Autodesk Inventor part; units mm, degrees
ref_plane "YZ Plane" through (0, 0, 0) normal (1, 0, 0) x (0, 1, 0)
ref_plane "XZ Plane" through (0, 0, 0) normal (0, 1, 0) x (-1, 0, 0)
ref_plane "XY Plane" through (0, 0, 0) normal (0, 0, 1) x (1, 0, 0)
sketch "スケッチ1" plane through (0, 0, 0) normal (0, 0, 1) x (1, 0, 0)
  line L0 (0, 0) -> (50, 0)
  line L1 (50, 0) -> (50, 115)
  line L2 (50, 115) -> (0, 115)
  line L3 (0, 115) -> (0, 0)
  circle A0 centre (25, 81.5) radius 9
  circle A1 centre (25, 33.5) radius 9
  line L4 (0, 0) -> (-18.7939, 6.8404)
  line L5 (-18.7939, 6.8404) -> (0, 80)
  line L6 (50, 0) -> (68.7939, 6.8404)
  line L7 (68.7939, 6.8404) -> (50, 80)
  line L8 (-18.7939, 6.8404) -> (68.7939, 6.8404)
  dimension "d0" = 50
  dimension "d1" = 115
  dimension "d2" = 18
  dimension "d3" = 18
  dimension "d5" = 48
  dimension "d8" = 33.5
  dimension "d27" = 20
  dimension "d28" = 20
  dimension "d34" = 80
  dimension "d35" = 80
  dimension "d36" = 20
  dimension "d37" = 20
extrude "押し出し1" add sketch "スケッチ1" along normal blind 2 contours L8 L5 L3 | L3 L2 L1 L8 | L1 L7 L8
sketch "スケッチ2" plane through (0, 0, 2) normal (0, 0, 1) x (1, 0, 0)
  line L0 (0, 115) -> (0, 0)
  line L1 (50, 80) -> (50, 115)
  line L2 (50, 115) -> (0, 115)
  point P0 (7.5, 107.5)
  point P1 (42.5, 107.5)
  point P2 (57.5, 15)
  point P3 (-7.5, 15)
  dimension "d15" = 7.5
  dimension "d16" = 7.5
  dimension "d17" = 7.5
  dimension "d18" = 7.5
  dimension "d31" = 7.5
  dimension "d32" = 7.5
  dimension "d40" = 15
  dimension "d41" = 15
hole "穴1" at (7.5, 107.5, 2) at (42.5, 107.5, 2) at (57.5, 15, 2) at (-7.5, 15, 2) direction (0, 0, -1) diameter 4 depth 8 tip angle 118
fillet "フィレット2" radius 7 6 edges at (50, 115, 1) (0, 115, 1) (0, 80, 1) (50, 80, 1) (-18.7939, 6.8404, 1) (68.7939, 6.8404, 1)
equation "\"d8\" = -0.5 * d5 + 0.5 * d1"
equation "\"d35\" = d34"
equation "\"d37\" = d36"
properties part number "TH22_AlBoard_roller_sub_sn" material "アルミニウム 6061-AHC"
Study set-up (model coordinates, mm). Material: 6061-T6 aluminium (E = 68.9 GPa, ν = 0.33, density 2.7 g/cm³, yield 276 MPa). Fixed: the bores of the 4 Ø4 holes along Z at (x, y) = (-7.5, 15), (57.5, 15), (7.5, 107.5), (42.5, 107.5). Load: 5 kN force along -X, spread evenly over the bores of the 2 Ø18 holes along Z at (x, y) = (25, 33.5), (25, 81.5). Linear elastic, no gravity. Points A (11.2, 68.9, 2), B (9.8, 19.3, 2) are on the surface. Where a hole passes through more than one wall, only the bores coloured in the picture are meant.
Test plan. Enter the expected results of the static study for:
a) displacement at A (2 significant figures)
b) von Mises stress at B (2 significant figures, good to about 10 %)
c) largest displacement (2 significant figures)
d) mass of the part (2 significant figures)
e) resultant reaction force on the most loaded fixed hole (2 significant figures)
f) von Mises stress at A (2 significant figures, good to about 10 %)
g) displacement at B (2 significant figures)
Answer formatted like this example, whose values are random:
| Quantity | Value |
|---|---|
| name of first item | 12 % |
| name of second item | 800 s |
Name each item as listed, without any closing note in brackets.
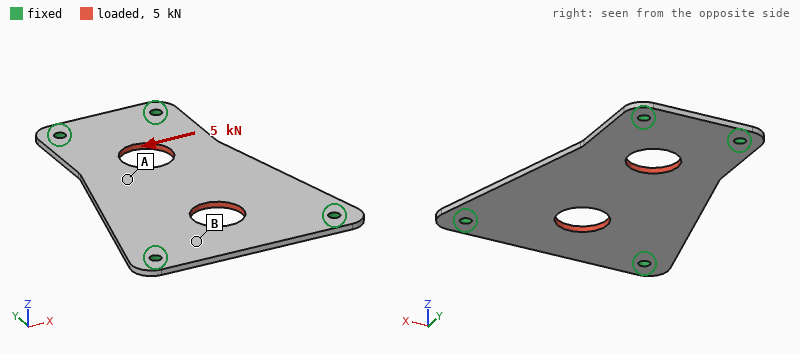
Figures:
| Quantity | Value |
|---|---|
| displacement at A | 40 µm |
| von Mises stress at B | 27 MPa |
| largest displacement | 42 µm |
| mass of the part | 33 g |
| resultant reaction force on the most loaded fixed hole | 1.8 kN |
| von Mises stress at A | 14 MPa |
| displacement at B | 11 µm |
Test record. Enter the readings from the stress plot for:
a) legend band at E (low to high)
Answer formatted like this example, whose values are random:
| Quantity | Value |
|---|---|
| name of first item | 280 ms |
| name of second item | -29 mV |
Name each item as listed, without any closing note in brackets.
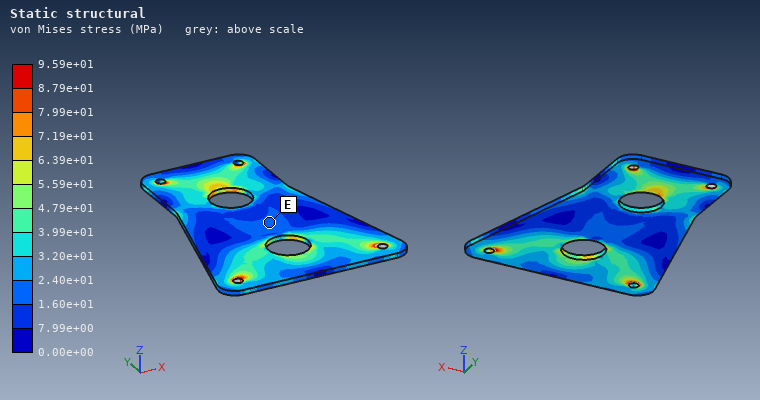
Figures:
| Quantity | Value |
|---|---|
| legend band at E | 1.60e+01 to 2.40e+01 MPa |
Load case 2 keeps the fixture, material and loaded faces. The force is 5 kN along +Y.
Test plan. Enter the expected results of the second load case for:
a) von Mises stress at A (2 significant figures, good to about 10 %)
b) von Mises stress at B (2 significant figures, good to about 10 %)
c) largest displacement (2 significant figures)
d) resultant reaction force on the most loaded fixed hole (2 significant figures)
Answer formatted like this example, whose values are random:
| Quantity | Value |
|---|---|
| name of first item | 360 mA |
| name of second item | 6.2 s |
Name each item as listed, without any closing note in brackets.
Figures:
| Quantity | Value |
|---|---|
| von Mises stress at A | 18 MPa |
| von Mises stress at B | 21 MPa |
| largest displacement | 28 µm |
| resultant reaction force on the most loaded fixed hole | 1.3 kN |
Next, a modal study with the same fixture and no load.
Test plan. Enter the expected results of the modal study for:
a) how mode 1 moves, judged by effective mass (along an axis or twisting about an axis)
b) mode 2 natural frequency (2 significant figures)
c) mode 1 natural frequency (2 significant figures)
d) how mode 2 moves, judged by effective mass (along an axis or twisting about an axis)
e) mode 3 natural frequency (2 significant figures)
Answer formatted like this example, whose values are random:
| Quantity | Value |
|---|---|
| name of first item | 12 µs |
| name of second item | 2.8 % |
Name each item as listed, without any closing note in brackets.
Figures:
| Quantity | Value |
|---|---|
| how mode 1 moves, judged by effective mass | along Z |
| mode 2 natural frequency | 1700 Hz |
| mode 1 natural frequency | 1100 Hz |
| how mode 2 moves, judged by effective mass | twisting about Y |
| mode 3 natural frequency | 2500 Hz |
